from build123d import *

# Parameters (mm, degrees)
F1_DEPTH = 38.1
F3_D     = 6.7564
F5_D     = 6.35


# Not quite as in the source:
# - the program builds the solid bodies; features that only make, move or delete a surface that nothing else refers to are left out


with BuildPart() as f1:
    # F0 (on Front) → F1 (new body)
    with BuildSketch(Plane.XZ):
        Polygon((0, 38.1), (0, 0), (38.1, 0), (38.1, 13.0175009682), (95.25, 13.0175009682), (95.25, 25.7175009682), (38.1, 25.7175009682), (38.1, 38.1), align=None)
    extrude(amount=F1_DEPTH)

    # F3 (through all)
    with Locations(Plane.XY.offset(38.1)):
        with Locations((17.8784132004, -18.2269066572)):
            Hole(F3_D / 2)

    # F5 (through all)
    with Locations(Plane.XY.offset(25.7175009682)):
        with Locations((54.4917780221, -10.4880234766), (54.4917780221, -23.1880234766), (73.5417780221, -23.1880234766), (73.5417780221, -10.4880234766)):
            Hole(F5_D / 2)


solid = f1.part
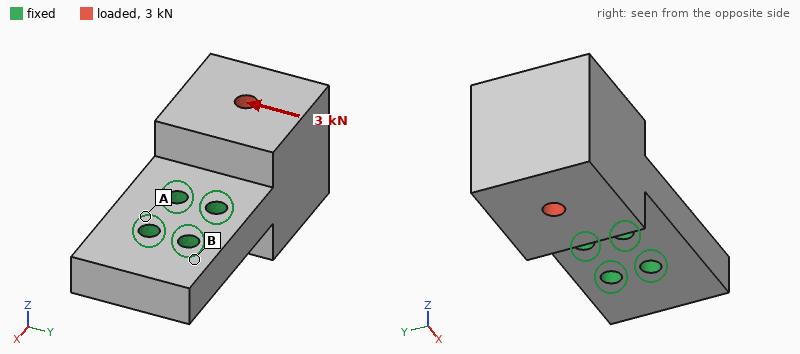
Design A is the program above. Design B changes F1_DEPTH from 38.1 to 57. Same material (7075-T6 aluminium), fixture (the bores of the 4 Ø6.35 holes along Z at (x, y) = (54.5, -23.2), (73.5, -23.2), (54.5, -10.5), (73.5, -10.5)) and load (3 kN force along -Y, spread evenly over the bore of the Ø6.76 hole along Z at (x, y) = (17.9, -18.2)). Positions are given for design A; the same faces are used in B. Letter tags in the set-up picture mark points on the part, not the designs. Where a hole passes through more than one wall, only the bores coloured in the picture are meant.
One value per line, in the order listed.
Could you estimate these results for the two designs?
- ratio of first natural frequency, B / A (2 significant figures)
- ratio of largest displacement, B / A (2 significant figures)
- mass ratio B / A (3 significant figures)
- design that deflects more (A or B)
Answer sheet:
0.88
0.68
1.51
A
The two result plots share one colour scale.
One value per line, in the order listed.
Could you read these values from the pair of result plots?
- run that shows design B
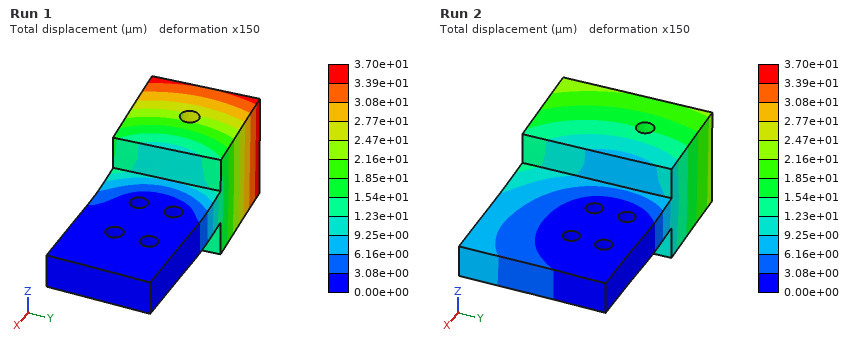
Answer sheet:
Run 2
